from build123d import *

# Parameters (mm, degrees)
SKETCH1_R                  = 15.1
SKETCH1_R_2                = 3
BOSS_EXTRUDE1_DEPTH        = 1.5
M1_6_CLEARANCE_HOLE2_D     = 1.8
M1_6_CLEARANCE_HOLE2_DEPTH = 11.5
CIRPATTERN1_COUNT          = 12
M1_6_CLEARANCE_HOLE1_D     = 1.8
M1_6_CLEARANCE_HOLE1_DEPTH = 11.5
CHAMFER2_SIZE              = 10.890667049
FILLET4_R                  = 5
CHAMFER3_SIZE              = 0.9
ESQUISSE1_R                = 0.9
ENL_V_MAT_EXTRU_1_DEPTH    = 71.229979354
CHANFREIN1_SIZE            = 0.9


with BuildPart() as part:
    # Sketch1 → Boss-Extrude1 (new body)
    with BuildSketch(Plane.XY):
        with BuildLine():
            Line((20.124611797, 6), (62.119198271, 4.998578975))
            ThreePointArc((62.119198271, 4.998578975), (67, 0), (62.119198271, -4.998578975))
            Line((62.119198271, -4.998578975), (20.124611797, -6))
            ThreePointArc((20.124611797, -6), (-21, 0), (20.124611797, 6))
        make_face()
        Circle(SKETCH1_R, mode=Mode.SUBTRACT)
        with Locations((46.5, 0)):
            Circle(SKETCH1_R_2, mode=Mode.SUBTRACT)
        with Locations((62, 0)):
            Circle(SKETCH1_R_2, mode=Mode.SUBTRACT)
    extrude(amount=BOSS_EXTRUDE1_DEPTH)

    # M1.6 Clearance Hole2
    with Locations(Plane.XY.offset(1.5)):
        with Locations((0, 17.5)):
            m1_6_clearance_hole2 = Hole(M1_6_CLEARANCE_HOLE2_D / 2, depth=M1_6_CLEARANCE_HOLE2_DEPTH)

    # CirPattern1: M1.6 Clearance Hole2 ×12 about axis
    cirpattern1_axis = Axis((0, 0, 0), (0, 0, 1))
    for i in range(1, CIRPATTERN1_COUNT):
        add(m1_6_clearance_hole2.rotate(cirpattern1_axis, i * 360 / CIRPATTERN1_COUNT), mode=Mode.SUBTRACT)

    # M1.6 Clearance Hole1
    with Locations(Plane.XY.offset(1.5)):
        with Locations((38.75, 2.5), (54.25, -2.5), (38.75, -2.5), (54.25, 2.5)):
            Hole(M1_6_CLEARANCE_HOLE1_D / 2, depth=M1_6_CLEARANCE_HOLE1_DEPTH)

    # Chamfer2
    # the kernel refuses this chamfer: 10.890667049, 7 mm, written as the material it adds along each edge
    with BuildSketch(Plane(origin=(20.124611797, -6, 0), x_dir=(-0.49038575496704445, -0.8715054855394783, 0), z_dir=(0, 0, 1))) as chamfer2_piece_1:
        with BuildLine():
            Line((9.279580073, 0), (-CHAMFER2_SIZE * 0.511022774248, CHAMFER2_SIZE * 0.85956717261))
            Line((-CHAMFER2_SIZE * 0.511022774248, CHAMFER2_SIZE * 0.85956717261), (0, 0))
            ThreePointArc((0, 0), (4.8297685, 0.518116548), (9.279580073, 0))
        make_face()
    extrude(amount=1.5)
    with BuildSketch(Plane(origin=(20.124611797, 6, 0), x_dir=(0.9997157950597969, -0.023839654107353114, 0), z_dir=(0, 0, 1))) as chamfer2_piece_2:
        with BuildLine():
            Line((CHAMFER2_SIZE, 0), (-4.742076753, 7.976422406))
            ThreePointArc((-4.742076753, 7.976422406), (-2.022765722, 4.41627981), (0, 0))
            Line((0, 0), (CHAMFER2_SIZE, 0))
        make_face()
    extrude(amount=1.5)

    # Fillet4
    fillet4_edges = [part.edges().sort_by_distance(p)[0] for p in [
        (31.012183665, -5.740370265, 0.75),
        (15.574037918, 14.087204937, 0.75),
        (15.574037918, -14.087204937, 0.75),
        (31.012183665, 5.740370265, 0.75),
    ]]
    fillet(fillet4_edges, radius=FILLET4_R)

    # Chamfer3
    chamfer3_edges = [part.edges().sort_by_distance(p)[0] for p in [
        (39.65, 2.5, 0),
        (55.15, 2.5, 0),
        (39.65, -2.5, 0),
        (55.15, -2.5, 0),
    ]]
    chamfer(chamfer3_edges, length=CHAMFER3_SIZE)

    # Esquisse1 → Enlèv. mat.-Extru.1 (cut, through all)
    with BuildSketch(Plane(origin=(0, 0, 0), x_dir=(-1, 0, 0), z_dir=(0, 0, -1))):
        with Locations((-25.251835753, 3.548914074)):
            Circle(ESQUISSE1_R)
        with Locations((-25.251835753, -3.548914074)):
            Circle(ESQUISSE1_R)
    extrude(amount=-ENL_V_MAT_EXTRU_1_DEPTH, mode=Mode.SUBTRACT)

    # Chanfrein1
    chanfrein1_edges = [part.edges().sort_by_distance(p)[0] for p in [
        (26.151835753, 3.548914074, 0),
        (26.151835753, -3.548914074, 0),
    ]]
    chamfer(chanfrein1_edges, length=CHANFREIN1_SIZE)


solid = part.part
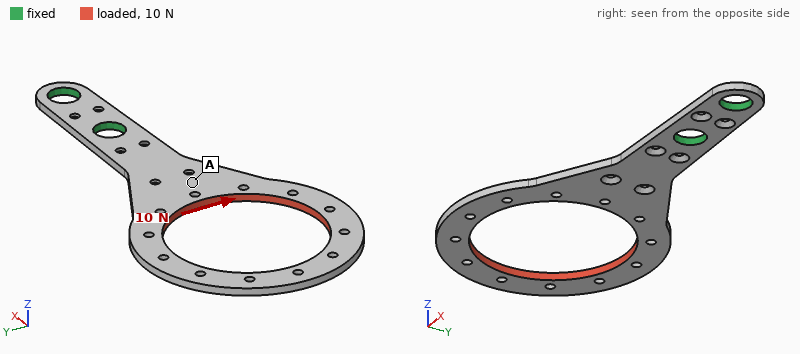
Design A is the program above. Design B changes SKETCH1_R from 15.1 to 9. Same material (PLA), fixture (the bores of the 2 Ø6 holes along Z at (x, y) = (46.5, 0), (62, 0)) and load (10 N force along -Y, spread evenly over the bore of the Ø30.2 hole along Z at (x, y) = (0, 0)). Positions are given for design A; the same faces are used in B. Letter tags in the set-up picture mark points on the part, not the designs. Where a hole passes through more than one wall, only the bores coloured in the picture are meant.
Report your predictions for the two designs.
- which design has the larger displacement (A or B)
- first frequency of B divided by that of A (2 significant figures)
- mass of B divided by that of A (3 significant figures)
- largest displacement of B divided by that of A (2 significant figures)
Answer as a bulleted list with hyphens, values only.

- A
- 0.81
- 1.41
- 0.86
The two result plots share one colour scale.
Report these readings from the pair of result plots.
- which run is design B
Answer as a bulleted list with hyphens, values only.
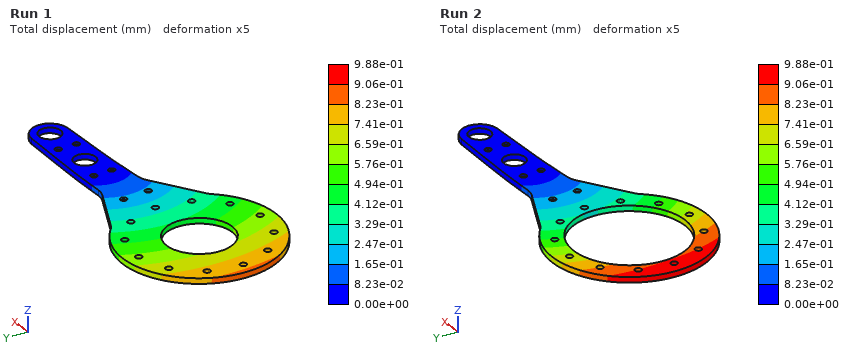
- Run 1
